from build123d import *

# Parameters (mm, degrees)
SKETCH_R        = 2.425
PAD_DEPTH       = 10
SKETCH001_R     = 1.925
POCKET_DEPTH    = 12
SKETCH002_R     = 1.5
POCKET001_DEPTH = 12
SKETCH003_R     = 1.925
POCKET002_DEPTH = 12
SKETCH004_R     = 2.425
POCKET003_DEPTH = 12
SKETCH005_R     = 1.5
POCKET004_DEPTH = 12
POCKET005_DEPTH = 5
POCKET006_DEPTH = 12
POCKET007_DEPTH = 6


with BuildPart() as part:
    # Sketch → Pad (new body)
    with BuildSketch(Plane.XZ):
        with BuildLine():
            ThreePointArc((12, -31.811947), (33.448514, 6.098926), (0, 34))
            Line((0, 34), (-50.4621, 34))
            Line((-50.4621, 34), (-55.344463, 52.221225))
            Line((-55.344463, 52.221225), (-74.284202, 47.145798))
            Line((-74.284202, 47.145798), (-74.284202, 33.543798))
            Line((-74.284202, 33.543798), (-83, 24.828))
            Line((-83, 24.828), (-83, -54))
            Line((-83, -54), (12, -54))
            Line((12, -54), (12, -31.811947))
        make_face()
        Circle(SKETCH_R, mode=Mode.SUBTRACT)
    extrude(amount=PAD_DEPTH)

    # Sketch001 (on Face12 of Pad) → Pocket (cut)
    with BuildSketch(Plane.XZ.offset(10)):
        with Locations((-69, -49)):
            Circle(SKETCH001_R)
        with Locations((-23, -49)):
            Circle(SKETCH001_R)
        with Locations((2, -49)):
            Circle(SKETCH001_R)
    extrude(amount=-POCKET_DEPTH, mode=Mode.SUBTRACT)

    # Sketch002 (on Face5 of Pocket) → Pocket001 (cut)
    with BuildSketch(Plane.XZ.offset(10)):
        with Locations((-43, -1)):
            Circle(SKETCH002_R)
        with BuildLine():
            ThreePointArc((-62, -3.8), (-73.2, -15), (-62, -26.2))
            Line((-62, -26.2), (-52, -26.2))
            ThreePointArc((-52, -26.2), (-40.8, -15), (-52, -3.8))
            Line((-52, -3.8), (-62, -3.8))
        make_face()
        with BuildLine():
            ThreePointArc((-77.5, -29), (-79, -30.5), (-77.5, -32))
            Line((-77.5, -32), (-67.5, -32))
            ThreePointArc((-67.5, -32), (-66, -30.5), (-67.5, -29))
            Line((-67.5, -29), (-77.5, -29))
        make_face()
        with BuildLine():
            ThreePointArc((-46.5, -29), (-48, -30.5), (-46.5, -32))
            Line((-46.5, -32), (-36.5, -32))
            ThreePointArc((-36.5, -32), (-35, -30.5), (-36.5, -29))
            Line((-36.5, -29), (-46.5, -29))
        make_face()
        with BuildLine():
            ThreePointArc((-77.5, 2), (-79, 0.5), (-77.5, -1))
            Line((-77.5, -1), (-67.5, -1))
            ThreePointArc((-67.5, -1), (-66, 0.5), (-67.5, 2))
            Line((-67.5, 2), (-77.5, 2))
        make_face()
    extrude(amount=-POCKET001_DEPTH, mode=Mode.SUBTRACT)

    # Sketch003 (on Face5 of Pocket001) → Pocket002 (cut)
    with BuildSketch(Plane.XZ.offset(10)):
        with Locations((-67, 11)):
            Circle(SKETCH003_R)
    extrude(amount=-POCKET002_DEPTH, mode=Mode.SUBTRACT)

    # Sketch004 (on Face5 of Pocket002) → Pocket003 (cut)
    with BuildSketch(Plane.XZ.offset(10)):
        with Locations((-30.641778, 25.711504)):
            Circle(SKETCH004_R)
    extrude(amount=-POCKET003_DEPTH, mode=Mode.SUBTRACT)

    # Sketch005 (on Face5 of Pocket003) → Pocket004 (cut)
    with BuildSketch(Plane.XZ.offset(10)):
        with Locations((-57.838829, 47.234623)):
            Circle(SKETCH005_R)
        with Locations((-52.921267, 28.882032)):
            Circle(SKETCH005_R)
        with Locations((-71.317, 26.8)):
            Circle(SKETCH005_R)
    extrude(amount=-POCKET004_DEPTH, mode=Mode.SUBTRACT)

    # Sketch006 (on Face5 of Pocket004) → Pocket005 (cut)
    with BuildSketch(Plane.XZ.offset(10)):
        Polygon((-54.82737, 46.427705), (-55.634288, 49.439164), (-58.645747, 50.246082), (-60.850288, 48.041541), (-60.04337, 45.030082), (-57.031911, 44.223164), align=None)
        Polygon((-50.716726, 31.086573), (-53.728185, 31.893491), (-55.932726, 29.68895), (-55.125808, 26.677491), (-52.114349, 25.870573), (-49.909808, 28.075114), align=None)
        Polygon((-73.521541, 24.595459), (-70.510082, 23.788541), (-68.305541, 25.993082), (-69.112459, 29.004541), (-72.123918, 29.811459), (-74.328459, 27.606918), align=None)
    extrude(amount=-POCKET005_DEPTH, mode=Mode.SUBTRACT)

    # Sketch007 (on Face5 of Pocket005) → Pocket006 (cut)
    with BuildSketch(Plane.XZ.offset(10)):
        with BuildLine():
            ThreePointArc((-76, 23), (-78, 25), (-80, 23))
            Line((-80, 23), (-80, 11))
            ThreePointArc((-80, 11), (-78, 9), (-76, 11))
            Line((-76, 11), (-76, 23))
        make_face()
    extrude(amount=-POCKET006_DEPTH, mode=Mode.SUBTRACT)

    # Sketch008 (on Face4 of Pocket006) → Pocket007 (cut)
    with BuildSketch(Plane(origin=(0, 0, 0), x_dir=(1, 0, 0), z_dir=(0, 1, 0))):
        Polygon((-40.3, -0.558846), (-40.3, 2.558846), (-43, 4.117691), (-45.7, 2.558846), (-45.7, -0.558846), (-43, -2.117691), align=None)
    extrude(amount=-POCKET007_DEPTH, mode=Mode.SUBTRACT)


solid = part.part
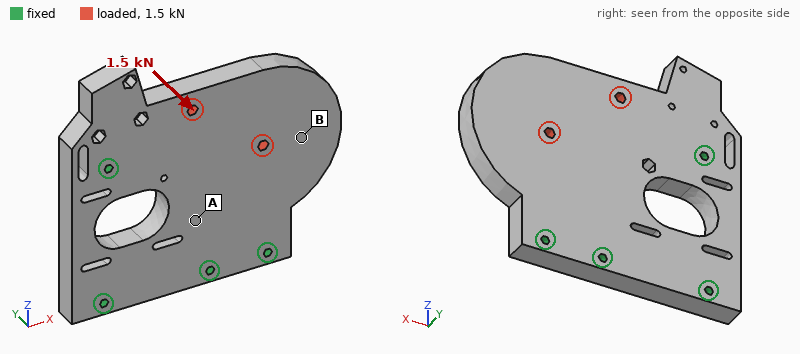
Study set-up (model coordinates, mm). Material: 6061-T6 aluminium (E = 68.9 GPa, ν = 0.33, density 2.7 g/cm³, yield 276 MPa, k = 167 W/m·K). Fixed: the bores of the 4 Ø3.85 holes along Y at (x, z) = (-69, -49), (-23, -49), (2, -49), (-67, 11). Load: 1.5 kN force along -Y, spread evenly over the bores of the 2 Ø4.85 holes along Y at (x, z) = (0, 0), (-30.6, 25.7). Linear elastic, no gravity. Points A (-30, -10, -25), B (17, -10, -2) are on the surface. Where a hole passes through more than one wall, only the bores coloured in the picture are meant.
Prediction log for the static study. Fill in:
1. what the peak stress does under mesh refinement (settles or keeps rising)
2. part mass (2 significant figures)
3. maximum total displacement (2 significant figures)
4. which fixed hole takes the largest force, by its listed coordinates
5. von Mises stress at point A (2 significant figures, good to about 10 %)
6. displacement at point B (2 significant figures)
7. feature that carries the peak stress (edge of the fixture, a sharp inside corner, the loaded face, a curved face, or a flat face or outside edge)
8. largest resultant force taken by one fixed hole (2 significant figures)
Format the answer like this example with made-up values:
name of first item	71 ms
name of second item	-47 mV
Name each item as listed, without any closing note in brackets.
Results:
what the peak stress does under mesh refinement	keeps rising
part mass	240 g
maximum total displacement	0.20 mm
which fixed hole takes the largest force, by its listed coordinates	(-67, 11)
von Mises stress at point A	19 MPa
displacement at point B	0.12 mm
feature that carries the peak stress	edge of the fixture
largest resultant force taken by one fixed hole	970 N
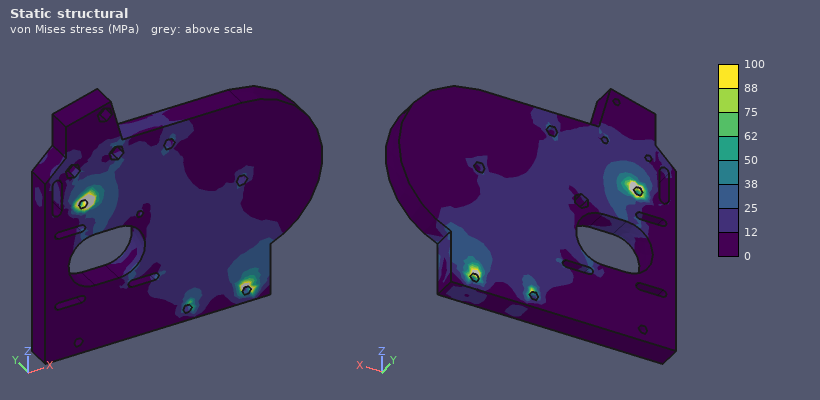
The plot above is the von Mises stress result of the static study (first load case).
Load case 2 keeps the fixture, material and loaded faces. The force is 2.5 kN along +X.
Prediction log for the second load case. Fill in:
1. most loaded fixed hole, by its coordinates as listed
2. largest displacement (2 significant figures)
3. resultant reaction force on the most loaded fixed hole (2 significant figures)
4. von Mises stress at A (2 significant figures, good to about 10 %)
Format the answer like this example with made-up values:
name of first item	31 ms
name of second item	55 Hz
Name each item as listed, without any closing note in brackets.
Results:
most loaded fixed hole, by its coordinates as listed	(-67, 11)
largest displacement	6.2 µm
resultant reaction force on the most loaded fixed hole	1.9 kN
von Mises stress at A	2.0 MPa
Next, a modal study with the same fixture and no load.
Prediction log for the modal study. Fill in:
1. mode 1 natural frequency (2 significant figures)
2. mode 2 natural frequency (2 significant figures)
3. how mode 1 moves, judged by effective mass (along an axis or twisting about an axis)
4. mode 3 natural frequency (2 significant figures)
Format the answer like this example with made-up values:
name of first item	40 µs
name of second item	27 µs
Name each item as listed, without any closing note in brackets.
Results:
mode 1 natural frequency	1600 Hz
mode 2 natural frequency	4500 Hz
how mode 1 moves, judged by effective mass	along Y
mode 3 natural frequency	6100 Hz
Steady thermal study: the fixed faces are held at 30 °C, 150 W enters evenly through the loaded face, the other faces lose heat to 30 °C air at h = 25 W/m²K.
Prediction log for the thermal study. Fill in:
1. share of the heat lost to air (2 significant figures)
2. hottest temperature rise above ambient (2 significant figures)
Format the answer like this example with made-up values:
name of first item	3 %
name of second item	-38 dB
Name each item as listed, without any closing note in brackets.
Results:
share of the heat lost to air	8.8 %
hottest temperature rise above ambient	58 K
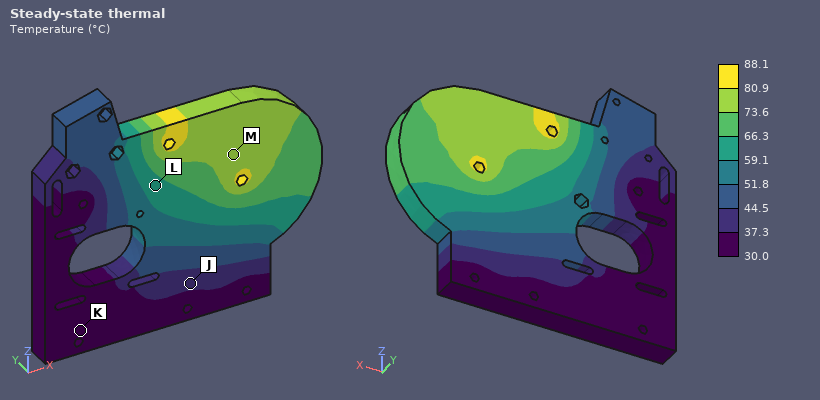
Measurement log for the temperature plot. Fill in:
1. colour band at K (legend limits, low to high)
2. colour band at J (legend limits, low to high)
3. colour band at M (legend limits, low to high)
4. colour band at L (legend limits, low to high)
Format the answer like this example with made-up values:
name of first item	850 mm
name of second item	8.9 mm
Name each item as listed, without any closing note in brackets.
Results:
colour band at K	30.0 to 37.3 °C
colour band at J	37.3 to 44.5 °C
colour band at M	73.6 to 80.9 °C
colour band at L	59.1 to 66.3 °C
